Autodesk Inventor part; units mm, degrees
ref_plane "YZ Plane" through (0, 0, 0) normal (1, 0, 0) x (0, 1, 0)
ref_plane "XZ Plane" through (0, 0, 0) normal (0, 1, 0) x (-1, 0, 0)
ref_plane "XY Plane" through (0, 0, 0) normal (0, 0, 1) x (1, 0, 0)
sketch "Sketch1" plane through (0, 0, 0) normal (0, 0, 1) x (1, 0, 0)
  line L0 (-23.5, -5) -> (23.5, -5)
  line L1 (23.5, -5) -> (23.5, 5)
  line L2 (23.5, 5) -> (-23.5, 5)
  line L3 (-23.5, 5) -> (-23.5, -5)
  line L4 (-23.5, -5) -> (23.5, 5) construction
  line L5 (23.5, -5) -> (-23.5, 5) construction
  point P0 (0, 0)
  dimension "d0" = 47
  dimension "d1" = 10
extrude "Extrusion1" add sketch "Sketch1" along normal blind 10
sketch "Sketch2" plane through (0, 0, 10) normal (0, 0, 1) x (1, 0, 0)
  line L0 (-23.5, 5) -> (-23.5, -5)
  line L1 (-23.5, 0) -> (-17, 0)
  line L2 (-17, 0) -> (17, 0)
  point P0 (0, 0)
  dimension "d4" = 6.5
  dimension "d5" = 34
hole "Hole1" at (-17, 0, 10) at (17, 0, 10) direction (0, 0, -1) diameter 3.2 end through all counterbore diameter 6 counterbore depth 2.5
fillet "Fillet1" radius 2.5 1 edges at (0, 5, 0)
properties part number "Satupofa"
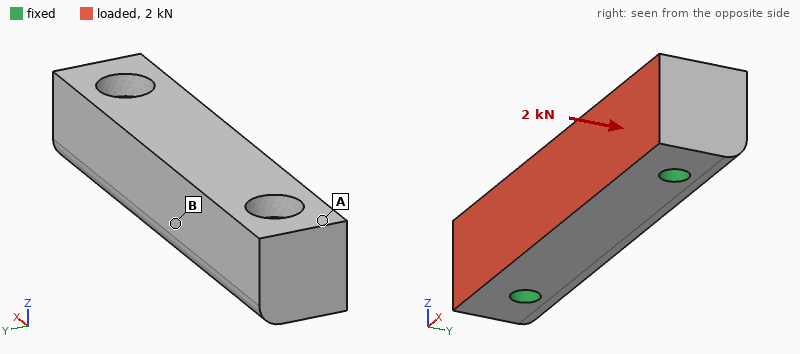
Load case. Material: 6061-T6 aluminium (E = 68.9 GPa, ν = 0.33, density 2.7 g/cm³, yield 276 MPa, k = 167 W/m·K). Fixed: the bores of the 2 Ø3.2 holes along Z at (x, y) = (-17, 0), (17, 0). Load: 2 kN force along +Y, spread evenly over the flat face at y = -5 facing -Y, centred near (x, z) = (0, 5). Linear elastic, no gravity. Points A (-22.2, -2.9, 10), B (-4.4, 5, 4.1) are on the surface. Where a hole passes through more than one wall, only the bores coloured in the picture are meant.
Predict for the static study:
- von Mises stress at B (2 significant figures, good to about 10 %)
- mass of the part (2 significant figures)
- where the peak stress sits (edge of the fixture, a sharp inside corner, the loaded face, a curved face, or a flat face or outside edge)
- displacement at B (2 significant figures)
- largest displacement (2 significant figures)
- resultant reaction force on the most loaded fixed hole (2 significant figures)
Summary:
16 MPa
12 g
edge of the fixture
6.6 µm
8.6 µm
1.0 kN
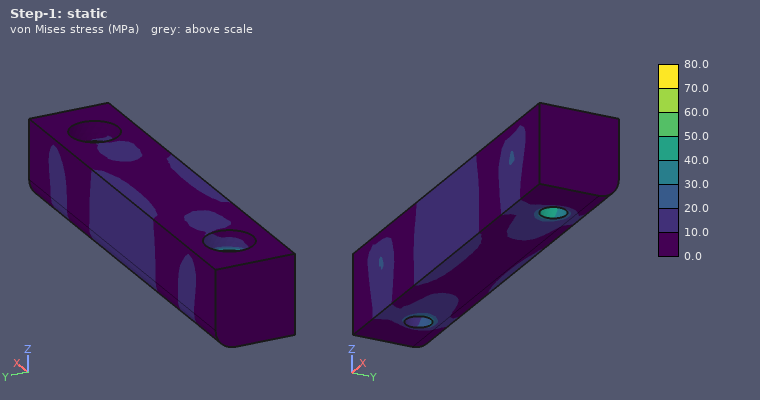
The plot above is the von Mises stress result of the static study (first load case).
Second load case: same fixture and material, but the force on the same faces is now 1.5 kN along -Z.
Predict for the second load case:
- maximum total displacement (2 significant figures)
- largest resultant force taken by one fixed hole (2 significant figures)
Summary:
11 µm
760 N
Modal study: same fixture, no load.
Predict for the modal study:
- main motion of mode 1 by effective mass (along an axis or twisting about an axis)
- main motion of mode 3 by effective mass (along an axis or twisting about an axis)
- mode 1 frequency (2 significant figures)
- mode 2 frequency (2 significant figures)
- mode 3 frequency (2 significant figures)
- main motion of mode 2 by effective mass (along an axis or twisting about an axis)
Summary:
along Y
twisting about X
24 kHz
28 kHz
38 kHz
along Z
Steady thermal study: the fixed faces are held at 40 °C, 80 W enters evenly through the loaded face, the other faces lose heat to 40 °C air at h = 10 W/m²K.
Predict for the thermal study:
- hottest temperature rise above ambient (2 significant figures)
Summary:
20 K
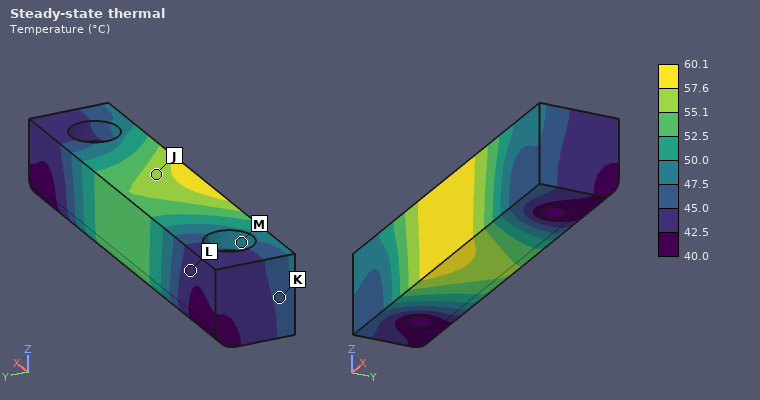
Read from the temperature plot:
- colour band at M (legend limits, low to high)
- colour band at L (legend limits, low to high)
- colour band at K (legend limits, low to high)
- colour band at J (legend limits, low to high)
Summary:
47.5 to 50.0 °C
42.5 to 45.0 °C
45.0 to 47.5 °C
55.1 to 57.6 °C
